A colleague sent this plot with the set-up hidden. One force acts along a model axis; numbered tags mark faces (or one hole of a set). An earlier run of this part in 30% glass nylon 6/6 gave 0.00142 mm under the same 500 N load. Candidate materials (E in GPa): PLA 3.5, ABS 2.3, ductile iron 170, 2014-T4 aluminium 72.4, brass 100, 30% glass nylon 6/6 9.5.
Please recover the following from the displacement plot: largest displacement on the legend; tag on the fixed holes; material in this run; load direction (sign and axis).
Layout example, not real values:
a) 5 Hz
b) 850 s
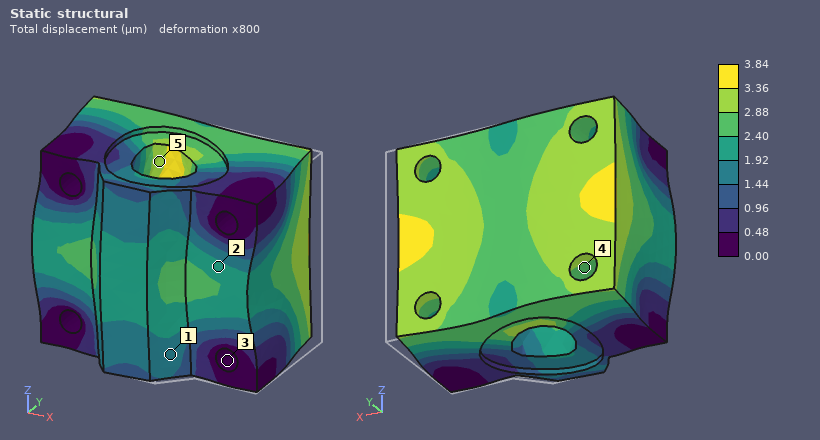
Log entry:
a) 3.84 µm
b) 3
c) PLA
d) -X
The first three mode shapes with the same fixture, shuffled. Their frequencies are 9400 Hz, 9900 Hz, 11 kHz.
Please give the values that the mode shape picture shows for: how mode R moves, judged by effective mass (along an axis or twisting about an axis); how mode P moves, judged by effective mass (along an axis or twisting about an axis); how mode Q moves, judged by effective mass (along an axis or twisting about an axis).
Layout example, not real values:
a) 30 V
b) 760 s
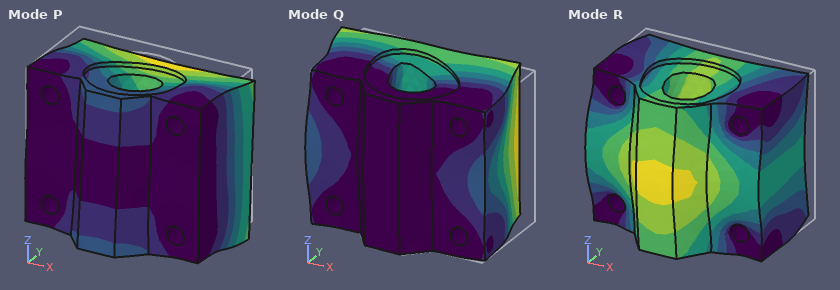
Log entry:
a) along Y
b) along Z
c) along X
